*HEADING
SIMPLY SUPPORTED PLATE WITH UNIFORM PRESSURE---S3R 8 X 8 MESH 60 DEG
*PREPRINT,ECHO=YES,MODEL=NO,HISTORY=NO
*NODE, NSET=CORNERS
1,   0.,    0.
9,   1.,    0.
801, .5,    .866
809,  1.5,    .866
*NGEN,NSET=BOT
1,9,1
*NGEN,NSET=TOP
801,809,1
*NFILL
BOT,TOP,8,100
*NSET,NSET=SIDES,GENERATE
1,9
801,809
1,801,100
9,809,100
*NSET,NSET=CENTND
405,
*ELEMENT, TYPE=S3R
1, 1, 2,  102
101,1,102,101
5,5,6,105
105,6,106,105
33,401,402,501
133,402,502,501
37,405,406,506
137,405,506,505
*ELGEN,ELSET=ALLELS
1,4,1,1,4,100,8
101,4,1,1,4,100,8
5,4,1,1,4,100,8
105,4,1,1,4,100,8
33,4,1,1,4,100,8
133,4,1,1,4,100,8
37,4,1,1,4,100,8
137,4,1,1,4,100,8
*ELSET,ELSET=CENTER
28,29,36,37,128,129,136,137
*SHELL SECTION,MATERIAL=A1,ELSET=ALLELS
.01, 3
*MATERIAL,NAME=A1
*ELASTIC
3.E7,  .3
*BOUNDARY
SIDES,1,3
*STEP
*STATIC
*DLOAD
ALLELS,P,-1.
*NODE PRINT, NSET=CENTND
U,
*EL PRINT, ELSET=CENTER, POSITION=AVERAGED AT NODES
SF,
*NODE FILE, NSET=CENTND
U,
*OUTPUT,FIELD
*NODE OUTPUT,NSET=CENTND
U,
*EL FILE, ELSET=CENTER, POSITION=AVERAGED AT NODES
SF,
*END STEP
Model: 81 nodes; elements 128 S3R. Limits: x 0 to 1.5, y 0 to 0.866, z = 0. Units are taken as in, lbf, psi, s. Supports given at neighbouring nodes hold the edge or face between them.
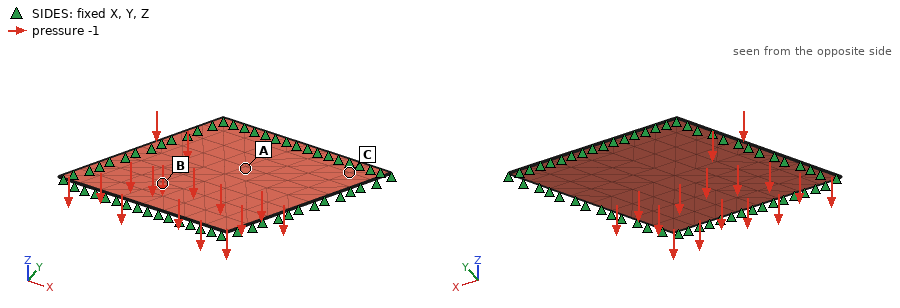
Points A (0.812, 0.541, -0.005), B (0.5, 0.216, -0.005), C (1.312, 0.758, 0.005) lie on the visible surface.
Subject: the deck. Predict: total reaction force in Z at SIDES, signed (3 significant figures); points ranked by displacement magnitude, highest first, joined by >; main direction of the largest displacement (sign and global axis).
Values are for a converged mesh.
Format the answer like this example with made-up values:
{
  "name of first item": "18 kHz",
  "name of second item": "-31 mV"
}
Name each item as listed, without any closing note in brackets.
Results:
{
  "total reaction force in Z at SIDES, signed": "0.866 lbf",
  "points ranked by displacement magnitude, highest first, joined by >": "A > B > C",
  "main direction of the largest displacement": "-Z"
}
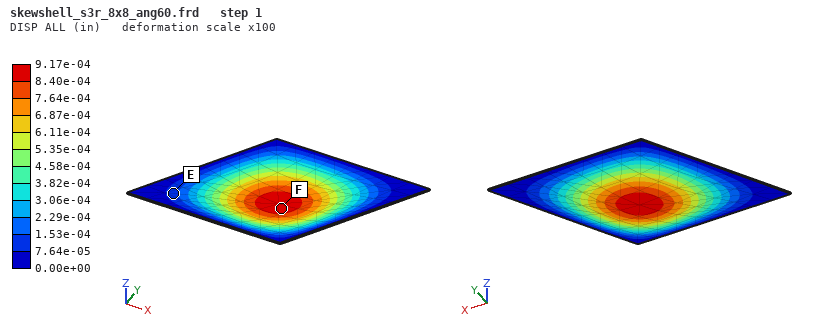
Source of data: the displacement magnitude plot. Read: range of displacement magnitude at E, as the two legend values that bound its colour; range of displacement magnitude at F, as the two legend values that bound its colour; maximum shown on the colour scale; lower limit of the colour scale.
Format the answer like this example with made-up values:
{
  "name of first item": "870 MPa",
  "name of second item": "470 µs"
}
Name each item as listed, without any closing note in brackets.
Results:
{
  "range of displacement magnitude at E, as the two legend values that bound its colour": "7.64e-05 to 1.53e-04 in",
  "range of displacement magnitude at F, as the two legend values that bound its colour": "8.40e-04 to 9.17e-04 in",
  "maximum shown on the colour scale": "9.17e-04 in",
  "lower limit of the colour scale": "0.00e+00 in"
}
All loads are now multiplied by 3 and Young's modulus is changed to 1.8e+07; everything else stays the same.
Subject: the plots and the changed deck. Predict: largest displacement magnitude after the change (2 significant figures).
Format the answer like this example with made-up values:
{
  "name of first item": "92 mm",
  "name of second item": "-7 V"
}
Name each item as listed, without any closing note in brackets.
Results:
{
  "largest displacement magnitude after the change": "0.0046 in"
}
